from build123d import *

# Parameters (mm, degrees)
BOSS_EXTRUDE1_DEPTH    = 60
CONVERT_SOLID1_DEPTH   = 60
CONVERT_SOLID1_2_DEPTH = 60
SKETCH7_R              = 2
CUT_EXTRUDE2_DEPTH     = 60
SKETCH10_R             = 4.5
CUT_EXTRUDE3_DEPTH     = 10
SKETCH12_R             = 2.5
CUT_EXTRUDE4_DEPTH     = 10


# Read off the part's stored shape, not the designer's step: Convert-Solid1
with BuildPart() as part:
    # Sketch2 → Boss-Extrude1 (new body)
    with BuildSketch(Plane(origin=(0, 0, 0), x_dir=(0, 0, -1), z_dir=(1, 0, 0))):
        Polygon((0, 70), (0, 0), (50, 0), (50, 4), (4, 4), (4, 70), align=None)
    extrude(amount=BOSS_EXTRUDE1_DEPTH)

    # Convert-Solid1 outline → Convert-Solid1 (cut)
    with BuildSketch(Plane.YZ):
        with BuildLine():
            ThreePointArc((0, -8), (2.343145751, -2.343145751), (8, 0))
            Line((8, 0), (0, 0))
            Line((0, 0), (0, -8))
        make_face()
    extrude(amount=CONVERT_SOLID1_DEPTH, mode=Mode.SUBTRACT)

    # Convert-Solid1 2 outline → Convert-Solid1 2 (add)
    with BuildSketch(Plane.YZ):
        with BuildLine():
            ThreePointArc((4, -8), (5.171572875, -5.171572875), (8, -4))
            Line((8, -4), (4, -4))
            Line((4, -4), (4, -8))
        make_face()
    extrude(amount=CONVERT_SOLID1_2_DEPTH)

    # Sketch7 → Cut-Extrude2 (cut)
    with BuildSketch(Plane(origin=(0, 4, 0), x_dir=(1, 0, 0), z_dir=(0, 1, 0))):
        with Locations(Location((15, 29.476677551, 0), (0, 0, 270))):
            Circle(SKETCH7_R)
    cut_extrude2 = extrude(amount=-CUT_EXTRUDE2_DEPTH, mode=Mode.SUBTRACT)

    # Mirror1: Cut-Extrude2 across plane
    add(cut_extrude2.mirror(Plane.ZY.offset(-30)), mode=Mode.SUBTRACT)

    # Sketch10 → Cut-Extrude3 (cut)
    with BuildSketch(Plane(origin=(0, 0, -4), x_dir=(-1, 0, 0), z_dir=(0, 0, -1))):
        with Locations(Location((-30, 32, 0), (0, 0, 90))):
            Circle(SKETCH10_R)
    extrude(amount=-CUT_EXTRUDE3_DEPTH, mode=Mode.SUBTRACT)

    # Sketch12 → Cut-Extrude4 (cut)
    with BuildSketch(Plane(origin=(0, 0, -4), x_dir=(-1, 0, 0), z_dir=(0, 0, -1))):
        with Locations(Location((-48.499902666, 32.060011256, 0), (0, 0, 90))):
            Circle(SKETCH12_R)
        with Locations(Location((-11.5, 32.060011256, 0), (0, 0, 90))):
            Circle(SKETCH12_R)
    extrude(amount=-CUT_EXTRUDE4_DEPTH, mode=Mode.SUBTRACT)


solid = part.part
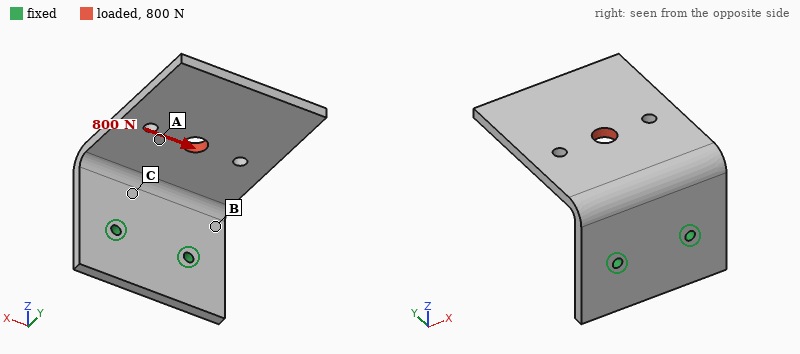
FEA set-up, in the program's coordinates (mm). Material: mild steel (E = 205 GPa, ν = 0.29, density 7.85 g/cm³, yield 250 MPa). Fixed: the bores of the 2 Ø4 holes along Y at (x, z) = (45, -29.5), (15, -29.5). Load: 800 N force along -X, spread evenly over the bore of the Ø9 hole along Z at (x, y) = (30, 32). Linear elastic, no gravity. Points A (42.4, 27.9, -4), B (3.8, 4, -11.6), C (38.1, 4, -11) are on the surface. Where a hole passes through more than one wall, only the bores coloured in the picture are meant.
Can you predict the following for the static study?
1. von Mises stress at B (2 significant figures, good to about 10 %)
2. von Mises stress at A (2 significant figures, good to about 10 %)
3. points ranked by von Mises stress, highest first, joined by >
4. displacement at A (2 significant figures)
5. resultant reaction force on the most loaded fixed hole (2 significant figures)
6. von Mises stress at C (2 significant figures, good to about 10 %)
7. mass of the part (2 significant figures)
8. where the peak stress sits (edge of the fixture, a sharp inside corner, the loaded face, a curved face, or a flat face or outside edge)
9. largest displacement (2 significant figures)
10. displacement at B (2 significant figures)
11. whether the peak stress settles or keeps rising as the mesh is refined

54 MPa
19 MPa
C > B > A
0.089 mm
1.0 kN
81 MPa
210 g
edge of the fixture
0.23 mm
0.050 mm
keeps rising
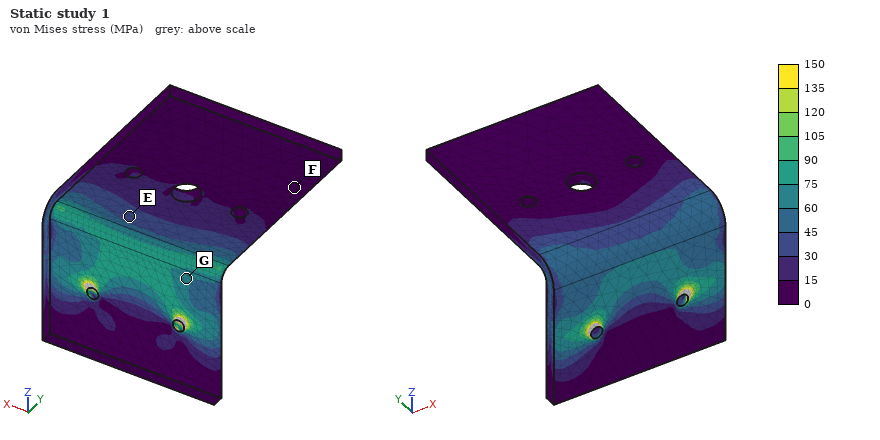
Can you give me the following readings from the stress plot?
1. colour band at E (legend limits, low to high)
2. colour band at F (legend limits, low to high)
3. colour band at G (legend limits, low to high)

30 to 45 MPa
0 to 15 MPa
60 to 75 MPa
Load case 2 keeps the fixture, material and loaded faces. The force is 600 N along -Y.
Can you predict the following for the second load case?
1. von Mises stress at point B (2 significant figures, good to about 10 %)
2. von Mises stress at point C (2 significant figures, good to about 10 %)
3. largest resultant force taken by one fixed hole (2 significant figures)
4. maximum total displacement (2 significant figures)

34 MPa
31 MPa
300 N
0.26 mm
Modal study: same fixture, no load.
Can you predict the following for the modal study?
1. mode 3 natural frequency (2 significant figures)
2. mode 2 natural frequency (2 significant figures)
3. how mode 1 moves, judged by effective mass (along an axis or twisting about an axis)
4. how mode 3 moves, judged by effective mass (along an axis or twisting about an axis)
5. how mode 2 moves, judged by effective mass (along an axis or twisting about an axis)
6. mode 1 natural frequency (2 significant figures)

1700 Hz
910 Hz
along Z
along Y
along X
440 Hz
